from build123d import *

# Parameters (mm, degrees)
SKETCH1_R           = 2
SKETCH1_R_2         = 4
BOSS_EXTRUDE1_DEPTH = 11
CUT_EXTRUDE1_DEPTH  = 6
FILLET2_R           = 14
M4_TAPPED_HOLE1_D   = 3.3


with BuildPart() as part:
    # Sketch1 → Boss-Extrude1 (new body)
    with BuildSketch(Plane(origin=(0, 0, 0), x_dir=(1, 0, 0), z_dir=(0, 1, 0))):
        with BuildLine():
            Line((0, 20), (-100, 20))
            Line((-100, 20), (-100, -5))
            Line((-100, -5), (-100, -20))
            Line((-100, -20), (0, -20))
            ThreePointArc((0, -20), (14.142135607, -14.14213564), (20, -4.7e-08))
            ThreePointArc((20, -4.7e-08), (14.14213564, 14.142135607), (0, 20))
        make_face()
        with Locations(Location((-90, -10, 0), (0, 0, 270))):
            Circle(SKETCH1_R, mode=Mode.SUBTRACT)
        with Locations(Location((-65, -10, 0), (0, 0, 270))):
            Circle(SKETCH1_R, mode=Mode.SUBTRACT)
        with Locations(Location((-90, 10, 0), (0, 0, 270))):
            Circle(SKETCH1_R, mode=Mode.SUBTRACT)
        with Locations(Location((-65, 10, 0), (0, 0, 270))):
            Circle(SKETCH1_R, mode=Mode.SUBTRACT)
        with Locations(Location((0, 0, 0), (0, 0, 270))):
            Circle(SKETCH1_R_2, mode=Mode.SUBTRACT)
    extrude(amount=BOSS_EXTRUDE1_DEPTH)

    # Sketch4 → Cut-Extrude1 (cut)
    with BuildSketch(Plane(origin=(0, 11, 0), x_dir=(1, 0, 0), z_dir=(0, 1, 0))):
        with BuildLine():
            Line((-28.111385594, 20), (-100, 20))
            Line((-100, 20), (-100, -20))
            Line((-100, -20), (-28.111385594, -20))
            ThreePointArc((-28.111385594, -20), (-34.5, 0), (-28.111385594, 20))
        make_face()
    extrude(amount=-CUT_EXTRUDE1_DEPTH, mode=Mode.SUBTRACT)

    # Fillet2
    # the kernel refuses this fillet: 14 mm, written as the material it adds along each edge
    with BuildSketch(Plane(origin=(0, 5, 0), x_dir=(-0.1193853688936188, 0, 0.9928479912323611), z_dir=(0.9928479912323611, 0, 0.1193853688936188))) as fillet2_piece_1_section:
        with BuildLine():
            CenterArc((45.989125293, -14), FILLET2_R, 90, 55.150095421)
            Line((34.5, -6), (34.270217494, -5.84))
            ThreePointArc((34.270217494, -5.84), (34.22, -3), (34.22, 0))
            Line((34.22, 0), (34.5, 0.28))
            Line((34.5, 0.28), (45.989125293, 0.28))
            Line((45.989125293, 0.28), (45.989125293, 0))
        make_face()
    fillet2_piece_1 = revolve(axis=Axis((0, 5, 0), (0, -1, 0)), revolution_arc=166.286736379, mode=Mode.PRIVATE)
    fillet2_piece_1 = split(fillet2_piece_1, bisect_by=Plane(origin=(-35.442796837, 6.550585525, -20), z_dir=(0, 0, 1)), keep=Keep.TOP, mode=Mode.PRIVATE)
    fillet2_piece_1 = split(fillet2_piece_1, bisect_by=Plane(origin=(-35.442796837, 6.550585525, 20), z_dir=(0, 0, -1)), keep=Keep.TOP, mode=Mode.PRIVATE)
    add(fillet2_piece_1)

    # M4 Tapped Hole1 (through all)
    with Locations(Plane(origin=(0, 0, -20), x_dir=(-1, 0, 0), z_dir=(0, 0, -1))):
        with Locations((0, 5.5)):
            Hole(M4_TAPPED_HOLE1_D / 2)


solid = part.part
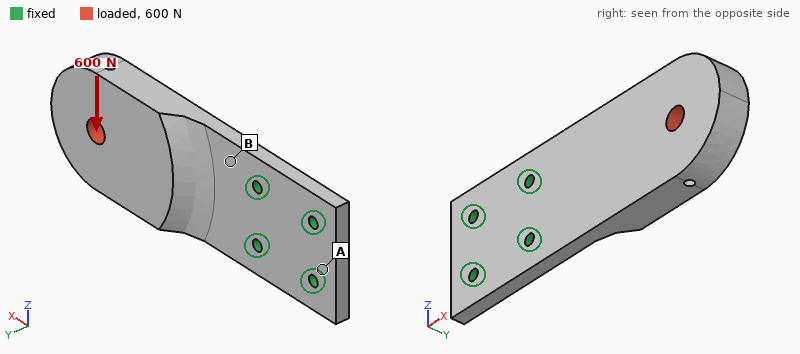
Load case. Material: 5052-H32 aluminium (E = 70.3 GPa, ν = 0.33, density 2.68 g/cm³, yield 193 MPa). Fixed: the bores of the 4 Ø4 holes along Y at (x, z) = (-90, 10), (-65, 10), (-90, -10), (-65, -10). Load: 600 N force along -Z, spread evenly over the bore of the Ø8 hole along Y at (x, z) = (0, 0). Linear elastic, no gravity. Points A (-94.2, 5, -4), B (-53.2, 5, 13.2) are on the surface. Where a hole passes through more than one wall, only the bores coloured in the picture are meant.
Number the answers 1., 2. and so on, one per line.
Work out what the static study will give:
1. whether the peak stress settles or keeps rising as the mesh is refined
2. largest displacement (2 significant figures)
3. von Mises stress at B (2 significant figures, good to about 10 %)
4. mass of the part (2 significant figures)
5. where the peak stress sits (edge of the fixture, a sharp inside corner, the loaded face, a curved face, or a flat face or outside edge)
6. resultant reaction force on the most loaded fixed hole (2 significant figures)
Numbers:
1. keeps rising
2. 57 µm
3. 19 MPa
4. 92 g
5. edge of the fixture
6. 1.3 kN
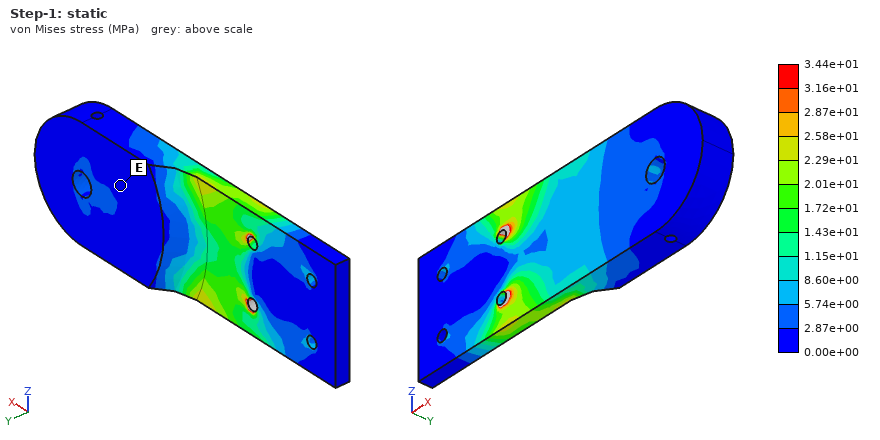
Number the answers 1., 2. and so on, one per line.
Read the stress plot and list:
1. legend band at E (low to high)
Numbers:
1. 0.00e+00 to 2.87e+00 MPa
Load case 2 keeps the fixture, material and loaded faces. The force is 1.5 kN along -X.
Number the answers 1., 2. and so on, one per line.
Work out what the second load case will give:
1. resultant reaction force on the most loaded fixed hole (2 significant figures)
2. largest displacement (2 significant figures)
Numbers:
1. 650 N
2. 0.28 mm
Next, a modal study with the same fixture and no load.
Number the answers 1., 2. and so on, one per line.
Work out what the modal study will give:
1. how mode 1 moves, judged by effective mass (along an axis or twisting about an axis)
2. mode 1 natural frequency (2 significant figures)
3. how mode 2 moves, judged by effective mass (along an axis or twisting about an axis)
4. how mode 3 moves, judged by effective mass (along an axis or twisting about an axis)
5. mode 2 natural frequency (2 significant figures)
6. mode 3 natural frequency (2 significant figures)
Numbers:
1. along Y
2. 490 Hz
3. along Z
4. along Z
5. 2600 Hz
6. 2900 Hz
